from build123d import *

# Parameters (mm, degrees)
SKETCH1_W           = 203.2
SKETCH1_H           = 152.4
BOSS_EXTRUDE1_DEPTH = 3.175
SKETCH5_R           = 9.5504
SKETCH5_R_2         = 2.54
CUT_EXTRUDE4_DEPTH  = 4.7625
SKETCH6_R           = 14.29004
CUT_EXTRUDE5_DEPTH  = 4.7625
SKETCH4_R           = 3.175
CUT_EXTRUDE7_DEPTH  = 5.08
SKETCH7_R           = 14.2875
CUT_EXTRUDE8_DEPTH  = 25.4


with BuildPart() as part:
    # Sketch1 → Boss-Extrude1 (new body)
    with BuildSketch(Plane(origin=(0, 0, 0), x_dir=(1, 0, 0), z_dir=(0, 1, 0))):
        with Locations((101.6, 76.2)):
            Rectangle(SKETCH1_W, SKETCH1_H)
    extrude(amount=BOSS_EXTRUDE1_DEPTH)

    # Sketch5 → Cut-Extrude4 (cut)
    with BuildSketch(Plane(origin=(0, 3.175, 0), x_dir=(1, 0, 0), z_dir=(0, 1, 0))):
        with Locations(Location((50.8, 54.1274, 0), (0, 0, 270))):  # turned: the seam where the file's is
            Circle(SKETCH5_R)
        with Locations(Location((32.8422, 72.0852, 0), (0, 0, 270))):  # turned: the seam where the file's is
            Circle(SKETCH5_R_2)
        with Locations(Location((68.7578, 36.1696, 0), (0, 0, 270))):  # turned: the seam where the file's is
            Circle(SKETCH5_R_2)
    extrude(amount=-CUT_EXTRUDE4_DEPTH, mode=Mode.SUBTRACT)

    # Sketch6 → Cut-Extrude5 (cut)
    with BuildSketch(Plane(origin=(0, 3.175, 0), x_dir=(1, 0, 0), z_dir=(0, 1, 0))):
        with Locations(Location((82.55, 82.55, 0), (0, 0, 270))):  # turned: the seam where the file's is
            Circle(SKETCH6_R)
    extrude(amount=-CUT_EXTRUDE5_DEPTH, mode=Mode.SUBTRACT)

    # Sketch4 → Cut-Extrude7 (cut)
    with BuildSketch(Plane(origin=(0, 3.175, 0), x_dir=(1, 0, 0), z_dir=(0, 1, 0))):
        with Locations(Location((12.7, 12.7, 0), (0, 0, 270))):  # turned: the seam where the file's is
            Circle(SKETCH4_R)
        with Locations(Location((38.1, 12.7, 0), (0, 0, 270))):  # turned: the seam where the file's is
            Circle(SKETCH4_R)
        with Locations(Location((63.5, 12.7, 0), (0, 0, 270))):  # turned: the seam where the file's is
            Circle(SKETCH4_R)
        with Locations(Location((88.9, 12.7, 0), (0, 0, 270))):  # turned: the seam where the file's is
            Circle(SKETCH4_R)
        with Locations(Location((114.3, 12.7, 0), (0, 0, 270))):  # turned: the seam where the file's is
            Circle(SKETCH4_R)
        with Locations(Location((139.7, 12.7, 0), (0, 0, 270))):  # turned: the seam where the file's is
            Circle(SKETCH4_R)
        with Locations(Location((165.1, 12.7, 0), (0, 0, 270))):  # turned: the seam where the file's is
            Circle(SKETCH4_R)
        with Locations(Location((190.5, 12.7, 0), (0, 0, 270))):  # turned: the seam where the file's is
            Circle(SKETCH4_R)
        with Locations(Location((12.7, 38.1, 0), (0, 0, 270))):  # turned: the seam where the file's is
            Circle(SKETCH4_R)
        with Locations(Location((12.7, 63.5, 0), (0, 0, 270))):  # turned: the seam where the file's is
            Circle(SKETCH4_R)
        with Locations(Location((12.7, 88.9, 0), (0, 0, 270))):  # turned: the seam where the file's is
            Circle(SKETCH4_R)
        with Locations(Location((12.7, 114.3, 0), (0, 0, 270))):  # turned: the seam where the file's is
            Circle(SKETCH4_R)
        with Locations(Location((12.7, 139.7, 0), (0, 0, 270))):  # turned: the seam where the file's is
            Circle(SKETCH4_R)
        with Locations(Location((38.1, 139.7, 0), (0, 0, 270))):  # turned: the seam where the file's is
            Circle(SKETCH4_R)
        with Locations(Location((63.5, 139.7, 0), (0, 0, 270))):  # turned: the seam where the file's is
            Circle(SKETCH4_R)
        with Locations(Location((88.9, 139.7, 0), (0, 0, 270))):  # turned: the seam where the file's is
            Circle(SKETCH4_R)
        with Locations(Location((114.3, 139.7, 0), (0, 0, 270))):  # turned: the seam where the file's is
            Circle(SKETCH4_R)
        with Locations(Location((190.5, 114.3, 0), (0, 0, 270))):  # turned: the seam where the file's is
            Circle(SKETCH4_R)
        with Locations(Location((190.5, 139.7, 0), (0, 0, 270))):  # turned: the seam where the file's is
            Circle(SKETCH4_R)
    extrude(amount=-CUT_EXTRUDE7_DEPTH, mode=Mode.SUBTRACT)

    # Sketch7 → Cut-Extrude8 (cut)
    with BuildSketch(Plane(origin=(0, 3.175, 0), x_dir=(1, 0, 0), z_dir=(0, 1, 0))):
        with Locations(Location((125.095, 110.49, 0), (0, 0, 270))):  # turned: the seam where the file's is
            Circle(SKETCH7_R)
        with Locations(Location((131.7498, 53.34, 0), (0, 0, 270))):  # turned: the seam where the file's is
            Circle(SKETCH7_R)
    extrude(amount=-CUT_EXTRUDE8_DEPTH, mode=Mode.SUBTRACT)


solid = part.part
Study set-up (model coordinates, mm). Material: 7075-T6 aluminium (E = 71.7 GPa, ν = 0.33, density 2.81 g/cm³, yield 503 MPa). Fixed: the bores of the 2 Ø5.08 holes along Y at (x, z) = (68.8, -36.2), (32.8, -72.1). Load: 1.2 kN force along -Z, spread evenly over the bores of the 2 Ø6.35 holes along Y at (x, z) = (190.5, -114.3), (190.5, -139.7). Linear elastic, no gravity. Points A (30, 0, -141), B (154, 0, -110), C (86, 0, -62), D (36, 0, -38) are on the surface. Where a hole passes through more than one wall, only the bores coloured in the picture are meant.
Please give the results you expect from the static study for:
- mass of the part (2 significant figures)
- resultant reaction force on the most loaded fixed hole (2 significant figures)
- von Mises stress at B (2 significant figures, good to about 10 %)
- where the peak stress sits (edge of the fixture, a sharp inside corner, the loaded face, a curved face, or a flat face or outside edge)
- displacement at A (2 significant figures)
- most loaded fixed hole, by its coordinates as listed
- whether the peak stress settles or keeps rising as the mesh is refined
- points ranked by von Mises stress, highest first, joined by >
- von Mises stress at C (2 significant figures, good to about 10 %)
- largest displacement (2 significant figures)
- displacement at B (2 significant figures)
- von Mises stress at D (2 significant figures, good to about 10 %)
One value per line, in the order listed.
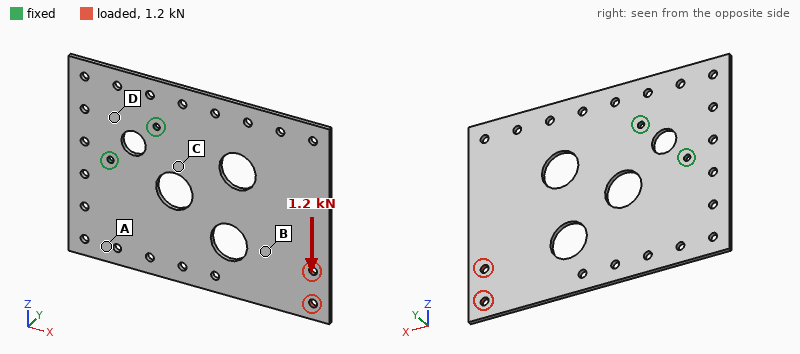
250 g
3.6 kN
8.8 MPa
edge of the fixture
0.061 mm
(68.8, -36.2)
keeps rising
C > D > B > A
22 MPa
0.16 mm
0.10 mm
15 MPa
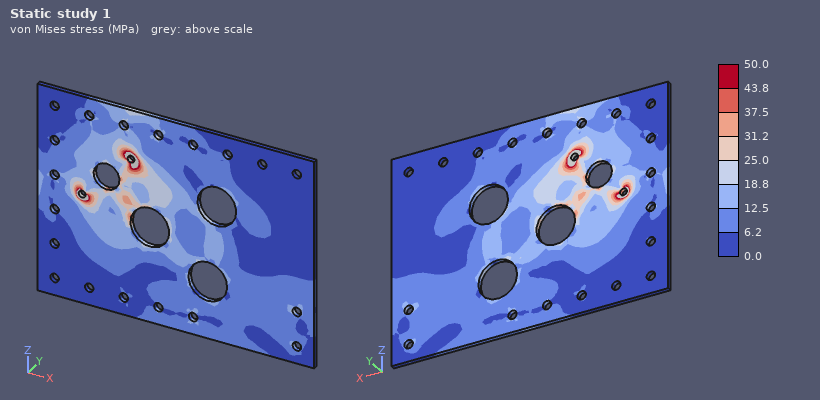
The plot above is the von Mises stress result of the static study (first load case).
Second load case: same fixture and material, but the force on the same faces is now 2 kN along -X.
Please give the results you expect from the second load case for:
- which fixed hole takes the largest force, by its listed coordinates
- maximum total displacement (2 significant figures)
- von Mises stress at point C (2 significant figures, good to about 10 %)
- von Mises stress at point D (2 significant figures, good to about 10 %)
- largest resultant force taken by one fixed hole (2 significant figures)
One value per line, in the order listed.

(32.8, -72.1)
0.15 mm
16 MPa
13 MPa
3.5 kN
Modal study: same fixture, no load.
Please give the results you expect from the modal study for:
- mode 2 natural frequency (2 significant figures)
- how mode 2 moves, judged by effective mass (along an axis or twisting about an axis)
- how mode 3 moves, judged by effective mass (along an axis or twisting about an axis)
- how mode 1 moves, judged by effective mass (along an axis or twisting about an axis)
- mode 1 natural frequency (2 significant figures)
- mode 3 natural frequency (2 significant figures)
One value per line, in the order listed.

210 Hz
twisting about X
along Y
along Y
100 Hz
410 Hz
